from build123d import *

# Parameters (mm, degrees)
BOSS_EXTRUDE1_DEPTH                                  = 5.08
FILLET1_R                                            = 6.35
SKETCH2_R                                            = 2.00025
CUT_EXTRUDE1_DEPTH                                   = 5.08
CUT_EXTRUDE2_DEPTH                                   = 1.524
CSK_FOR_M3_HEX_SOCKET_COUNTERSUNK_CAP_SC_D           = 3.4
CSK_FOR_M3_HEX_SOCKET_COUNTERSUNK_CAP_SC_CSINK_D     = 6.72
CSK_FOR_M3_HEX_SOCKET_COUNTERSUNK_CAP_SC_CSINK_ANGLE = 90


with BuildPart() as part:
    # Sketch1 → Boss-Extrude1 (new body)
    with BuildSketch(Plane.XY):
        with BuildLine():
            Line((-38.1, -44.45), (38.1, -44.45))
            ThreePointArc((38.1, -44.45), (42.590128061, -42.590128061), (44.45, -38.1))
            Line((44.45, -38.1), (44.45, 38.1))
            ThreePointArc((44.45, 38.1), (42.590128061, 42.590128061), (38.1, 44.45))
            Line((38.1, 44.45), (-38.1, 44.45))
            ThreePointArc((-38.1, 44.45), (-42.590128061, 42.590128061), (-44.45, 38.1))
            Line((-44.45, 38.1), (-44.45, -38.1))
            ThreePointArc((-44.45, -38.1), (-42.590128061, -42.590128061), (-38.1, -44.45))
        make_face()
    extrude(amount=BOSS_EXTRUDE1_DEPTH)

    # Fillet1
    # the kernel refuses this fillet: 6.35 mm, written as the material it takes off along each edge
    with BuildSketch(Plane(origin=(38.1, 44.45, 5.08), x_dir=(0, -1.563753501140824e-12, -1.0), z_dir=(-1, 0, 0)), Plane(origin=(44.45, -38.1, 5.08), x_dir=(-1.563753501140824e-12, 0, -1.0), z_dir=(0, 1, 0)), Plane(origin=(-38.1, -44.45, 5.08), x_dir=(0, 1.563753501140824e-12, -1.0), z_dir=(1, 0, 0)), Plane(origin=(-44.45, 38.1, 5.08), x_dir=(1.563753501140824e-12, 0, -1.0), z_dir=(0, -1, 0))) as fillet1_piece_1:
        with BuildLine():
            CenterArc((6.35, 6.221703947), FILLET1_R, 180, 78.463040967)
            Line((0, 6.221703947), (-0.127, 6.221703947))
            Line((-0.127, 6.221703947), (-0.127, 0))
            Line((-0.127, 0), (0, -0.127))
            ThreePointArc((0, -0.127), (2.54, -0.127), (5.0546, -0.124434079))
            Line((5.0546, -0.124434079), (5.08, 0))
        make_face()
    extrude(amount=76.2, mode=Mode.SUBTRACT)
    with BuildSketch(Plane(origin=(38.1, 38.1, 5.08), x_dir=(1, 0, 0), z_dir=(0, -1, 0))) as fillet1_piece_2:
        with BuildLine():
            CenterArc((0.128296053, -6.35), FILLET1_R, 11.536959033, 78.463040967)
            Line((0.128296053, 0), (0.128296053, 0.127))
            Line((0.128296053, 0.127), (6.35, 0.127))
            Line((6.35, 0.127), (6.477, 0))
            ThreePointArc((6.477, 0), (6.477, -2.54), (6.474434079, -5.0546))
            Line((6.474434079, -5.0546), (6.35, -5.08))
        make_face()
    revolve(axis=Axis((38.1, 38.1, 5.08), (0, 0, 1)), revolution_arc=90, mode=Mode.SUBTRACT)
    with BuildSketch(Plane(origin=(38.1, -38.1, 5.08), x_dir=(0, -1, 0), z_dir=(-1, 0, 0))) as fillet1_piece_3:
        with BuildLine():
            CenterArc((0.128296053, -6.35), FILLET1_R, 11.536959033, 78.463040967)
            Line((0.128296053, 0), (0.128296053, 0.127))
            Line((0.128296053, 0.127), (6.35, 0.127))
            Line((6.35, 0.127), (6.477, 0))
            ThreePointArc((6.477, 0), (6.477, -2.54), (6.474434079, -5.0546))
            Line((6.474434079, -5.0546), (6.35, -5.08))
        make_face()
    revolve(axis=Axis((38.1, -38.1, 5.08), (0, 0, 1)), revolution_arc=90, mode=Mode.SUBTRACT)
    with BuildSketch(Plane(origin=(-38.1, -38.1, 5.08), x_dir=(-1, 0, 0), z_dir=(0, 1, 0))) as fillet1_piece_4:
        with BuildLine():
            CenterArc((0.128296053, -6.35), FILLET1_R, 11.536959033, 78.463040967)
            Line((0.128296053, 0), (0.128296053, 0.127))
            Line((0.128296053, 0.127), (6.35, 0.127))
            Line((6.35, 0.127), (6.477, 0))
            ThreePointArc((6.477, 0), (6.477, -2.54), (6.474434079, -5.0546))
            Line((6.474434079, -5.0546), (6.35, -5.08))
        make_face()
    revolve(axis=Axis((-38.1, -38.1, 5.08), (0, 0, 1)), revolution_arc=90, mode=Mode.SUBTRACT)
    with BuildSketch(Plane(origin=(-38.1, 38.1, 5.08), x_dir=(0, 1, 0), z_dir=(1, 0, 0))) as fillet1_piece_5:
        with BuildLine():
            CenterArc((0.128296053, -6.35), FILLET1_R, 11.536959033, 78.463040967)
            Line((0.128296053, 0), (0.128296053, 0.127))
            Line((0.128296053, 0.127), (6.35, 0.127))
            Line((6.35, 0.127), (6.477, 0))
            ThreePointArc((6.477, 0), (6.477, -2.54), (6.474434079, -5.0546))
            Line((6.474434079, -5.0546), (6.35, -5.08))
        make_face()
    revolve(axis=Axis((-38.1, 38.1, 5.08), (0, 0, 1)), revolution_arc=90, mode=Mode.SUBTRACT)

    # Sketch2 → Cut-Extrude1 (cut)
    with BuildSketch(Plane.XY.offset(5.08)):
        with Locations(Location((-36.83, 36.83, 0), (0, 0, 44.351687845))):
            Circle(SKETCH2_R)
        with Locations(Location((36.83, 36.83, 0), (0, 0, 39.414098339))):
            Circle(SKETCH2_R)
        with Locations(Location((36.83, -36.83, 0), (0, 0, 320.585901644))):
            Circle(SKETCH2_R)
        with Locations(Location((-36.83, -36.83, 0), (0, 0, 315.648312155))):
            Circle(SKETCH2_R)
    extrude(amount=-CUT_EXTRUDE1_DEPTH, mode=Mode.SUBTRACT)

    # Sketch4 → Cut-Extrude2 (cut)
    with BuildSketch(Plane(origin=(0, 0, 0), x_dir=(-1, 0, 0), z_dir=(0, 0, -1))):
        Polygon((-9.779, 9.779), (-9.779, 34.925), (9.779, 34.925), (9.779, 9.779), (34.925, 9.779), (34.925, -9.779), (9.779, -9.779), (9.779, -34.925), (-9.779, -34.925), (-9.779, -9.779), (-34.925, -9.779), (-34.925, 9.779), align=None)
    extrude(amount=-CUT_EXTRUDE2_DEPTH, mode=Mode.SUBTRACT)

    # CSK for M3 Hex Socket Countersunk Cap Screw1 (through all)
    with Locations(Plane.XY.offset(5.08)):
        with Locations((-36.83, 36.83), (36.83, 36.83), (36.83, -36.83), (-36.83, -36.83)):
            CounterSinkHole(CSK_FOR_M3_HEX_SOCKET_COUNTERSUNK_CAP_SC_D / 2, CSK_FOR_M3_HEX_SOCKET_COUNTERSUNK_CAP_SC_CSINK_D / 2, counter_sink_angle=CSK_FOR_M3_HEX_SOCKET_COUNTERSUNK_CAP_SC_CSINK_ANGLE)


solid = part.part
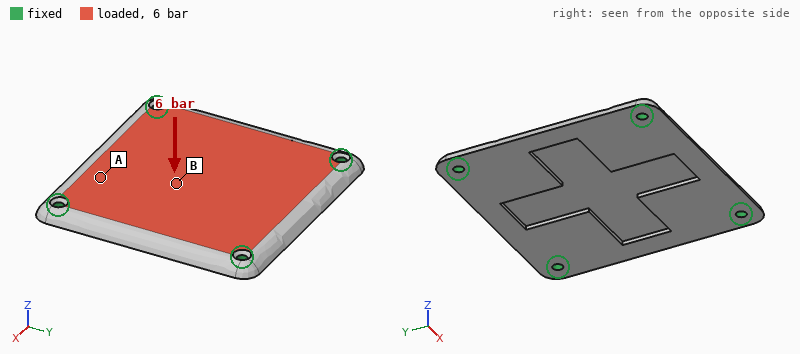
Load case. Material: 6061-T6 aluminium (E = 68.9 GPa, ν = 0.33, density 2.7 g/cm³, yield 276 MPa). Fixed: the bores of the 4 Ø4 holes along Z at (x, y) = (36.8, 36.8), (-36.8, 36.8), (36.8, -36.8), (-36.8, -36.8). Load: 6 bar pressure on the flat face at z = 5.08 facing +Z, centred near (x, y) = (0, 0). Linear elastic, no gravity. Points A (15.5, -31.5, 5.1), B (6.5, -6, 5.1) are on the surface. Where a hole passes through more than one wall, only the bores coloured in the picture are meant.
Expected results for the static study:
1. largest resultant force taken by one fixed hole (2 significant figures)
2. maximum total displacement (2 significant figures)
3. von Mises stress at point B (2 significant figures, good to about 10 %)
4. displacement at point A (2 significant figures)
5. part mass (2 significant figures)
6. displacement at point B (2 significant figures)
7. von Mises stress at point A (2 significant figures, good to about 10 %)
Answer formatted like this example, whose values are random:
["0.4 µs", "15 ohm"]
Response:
["1.5 kN", "0.28 mm", "68 MPa", "0.11 mm", "90 g", "0.26 mm", "26 MPa"]
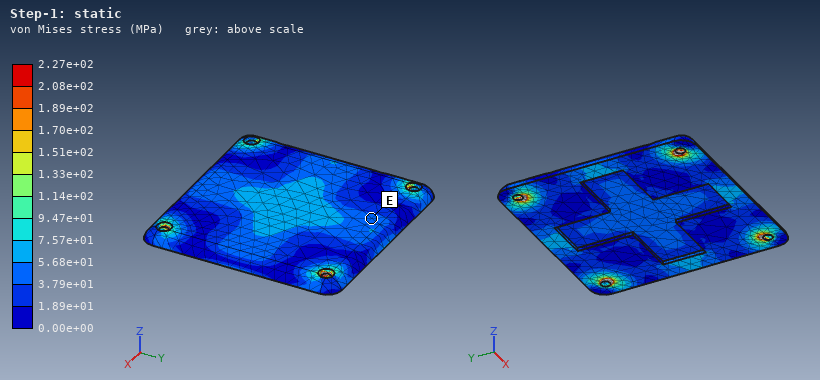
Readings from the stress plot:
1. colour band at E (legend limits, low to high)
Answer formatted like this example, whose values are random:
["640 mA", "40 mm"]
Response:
["3.79e+01 to 5.68e+01 MPa"]
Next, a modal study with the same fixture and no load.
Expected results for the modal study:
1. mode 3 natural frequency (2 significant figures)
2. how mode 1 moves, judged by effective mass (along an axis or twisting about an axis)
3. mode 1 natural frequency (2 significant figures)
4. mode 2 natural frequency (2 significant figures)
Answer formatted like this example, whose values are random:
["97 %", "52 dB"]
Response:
["4600 Hz", "along Z", "2700 Hz", "4600 Hz"]
